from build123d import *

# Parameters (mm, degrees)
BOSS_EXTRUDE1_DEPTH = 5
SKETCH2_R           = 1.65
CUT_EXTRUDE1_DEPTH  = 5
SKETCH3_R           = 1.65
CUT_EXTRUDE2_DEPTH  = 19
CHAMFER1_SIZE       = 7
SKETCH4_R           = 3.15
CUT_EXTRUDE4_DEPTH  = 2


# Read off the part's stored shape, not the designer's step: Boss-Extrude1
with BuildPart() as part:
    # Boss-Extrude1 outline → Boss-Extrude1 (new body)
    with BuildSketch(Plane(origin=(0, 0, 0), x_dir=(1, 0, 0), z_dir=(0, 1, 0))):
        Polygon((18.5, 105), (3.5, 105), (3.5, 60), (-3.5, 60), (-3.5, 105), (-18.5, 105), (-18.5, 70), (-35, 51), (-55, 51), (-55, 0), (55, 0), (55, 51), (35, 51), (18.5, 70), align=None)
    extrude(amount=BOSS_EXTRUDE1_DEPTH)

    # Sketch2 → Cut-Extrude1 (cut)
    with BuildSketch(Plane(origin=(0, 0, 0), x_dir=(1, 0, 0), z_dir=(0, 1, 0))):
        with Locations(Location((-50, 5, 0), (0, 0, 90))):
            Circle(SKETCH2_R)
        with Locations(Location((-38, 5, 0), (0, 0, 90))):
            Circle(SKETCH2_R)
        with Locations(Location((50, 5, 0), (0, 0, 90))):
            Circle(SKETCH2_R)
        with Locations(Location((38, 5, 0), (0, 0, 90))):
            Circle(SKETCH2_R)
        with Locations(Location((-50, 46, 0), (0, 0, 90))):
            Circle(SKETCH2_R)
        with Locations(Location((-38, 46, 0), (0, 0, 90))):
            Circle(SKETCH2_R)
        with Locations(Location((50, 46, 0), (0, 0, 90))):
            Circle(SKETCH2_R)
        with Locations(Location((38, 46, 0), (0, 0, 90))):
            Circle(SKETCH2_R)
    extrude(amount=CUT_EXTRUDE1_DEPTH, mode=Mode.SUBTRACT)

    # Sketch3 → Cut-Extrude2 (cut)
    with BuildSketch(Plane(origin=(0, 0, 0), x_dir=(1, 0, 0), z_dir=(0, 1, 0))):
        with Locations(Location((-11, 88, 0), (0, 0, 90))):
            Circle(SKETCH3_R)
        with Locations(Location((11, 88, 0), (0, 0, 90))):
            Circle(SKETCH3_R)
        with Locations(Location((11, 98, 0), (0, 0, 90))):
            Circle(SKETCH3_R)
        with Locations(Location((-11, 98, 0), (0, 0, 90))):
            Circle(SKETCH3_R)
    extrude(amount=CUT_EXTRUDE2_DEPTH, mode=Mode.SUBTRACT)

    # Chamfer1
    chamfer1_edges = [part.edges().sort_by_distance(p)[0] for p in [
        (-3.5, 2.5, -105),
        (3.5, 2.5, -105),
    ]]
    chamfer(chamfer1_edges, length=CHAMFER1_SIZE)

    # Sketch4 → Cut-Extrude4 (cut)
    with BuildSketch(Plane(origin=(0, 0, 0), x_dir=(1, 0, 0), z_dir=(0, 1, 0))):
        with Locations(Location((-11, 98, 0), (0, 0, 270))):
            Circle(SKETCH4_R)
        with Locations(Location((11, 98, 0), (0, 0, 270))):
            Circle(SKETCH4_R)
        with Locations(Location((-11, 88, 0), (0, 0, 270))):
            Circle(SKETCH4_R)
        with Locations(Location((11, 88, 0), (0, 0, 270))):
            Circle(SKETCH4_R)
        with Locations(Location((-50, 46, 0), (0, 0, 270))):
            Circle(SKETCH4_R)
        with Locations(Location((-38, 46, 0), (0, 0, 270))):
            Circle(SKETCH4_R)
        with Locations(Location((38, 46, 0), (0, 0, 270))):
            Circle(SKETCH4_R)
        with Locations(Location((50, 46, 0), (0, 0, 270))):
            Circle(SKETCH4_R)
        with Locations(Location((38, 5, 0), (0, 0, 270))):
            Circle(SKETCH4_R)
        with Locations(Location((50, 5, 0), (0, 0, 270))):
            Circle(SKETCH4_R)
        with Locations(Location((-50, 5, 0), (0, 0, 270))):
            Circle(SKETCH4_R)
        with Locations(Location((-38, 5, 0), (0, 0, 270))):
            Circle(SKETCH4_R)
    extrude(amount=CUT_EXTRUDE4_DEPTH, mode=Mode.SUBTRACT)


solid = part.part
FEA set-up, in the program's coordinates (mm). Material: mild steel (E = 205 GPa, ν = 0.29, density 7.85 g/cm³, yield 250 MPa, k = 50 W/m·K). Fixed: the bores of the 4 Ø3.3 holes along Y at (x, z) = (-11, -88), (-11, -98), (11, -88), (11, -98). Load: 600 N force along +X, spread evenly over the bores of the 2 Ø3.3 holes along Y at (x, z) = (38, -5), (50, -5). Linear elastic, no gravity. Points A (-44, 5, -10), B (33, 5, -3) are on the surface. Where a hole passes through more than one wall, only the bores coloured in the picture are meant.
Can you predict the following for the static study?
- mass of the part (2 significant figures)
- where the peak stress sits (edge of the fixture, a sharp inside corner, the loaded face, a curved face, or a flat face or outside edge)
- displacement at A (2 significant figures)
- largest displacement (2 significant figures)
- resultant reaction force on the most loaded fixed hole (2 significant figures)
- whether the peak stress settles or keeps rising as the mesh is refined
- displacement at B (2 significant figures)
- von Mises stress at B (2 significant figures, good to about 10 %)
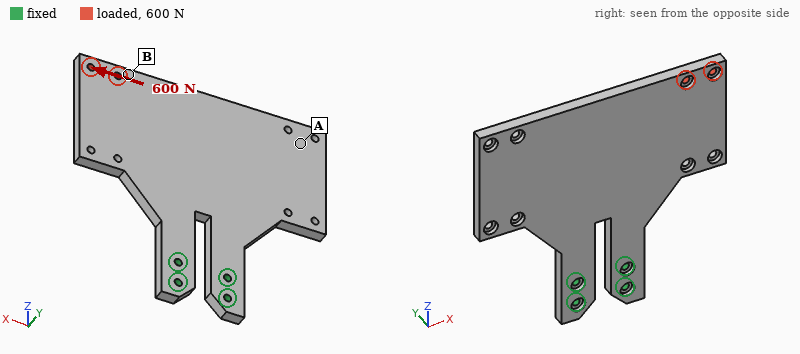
290 g
edge of the fixture
43 µm
56 µm
1.5 kN
keeps rising
45 µm
15 MPa
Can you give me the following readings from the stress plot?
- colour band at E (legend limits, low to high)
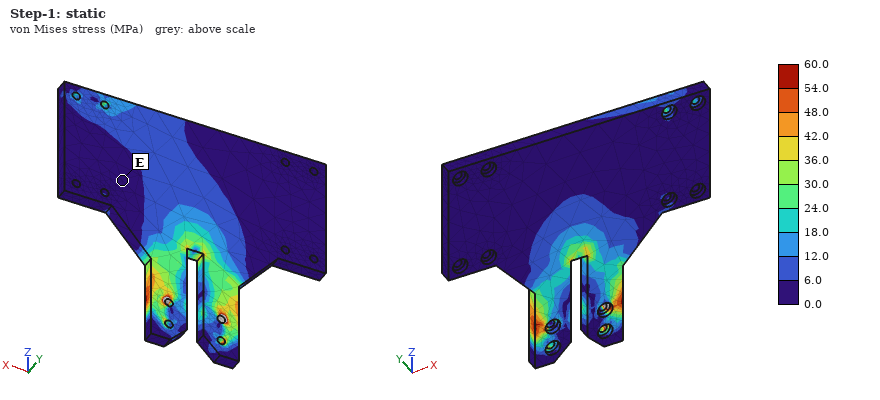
0.0 to 6.0 MPa
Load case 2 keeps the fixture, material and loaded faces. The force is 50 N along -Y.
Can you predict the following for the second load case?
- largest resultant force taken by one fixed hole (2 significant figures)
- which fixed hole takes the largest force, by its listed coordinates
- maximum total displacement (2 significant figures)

260 N
(11, -88)
0.21 mm
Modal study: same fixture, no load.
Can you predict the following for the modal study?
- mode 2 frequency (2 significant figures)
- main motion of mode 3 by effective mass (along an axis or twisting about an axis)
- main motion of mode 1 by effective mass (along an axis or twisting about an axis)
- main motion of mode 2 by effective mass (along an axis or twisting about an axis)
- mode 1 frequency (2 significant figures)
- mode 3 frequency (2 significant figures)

550 Hz
along X
along Y
twisting about Z
280 Hz
1600 Hz
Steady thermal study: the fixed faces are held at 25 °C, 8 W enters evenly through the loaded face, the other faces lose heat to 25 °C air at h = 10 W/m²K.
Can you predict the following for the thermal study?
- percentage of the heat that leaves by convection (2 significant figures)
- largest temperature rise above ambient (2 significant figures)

49 %
62 K
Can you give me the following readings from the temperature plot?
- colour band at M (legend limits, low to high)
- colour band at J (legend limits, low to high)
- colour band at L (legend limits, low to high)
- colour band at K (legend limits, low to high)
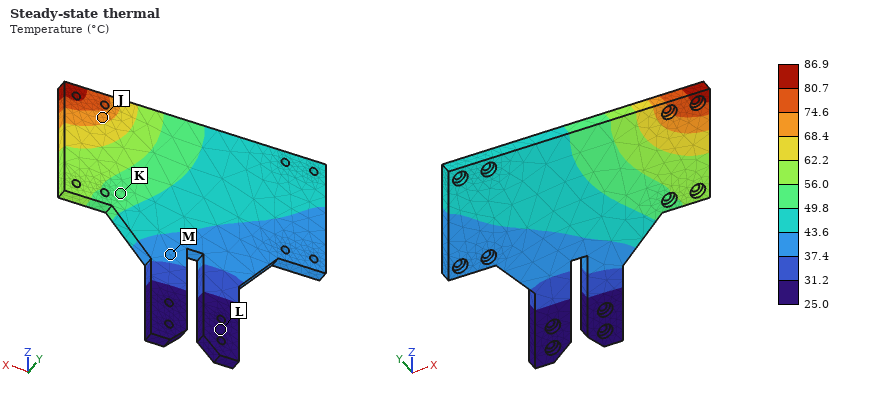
37.4 to 43.6 °C
68.4 to 74.6 °C
25.0 to 31.2 °C
49.8 to 56.0 °C
